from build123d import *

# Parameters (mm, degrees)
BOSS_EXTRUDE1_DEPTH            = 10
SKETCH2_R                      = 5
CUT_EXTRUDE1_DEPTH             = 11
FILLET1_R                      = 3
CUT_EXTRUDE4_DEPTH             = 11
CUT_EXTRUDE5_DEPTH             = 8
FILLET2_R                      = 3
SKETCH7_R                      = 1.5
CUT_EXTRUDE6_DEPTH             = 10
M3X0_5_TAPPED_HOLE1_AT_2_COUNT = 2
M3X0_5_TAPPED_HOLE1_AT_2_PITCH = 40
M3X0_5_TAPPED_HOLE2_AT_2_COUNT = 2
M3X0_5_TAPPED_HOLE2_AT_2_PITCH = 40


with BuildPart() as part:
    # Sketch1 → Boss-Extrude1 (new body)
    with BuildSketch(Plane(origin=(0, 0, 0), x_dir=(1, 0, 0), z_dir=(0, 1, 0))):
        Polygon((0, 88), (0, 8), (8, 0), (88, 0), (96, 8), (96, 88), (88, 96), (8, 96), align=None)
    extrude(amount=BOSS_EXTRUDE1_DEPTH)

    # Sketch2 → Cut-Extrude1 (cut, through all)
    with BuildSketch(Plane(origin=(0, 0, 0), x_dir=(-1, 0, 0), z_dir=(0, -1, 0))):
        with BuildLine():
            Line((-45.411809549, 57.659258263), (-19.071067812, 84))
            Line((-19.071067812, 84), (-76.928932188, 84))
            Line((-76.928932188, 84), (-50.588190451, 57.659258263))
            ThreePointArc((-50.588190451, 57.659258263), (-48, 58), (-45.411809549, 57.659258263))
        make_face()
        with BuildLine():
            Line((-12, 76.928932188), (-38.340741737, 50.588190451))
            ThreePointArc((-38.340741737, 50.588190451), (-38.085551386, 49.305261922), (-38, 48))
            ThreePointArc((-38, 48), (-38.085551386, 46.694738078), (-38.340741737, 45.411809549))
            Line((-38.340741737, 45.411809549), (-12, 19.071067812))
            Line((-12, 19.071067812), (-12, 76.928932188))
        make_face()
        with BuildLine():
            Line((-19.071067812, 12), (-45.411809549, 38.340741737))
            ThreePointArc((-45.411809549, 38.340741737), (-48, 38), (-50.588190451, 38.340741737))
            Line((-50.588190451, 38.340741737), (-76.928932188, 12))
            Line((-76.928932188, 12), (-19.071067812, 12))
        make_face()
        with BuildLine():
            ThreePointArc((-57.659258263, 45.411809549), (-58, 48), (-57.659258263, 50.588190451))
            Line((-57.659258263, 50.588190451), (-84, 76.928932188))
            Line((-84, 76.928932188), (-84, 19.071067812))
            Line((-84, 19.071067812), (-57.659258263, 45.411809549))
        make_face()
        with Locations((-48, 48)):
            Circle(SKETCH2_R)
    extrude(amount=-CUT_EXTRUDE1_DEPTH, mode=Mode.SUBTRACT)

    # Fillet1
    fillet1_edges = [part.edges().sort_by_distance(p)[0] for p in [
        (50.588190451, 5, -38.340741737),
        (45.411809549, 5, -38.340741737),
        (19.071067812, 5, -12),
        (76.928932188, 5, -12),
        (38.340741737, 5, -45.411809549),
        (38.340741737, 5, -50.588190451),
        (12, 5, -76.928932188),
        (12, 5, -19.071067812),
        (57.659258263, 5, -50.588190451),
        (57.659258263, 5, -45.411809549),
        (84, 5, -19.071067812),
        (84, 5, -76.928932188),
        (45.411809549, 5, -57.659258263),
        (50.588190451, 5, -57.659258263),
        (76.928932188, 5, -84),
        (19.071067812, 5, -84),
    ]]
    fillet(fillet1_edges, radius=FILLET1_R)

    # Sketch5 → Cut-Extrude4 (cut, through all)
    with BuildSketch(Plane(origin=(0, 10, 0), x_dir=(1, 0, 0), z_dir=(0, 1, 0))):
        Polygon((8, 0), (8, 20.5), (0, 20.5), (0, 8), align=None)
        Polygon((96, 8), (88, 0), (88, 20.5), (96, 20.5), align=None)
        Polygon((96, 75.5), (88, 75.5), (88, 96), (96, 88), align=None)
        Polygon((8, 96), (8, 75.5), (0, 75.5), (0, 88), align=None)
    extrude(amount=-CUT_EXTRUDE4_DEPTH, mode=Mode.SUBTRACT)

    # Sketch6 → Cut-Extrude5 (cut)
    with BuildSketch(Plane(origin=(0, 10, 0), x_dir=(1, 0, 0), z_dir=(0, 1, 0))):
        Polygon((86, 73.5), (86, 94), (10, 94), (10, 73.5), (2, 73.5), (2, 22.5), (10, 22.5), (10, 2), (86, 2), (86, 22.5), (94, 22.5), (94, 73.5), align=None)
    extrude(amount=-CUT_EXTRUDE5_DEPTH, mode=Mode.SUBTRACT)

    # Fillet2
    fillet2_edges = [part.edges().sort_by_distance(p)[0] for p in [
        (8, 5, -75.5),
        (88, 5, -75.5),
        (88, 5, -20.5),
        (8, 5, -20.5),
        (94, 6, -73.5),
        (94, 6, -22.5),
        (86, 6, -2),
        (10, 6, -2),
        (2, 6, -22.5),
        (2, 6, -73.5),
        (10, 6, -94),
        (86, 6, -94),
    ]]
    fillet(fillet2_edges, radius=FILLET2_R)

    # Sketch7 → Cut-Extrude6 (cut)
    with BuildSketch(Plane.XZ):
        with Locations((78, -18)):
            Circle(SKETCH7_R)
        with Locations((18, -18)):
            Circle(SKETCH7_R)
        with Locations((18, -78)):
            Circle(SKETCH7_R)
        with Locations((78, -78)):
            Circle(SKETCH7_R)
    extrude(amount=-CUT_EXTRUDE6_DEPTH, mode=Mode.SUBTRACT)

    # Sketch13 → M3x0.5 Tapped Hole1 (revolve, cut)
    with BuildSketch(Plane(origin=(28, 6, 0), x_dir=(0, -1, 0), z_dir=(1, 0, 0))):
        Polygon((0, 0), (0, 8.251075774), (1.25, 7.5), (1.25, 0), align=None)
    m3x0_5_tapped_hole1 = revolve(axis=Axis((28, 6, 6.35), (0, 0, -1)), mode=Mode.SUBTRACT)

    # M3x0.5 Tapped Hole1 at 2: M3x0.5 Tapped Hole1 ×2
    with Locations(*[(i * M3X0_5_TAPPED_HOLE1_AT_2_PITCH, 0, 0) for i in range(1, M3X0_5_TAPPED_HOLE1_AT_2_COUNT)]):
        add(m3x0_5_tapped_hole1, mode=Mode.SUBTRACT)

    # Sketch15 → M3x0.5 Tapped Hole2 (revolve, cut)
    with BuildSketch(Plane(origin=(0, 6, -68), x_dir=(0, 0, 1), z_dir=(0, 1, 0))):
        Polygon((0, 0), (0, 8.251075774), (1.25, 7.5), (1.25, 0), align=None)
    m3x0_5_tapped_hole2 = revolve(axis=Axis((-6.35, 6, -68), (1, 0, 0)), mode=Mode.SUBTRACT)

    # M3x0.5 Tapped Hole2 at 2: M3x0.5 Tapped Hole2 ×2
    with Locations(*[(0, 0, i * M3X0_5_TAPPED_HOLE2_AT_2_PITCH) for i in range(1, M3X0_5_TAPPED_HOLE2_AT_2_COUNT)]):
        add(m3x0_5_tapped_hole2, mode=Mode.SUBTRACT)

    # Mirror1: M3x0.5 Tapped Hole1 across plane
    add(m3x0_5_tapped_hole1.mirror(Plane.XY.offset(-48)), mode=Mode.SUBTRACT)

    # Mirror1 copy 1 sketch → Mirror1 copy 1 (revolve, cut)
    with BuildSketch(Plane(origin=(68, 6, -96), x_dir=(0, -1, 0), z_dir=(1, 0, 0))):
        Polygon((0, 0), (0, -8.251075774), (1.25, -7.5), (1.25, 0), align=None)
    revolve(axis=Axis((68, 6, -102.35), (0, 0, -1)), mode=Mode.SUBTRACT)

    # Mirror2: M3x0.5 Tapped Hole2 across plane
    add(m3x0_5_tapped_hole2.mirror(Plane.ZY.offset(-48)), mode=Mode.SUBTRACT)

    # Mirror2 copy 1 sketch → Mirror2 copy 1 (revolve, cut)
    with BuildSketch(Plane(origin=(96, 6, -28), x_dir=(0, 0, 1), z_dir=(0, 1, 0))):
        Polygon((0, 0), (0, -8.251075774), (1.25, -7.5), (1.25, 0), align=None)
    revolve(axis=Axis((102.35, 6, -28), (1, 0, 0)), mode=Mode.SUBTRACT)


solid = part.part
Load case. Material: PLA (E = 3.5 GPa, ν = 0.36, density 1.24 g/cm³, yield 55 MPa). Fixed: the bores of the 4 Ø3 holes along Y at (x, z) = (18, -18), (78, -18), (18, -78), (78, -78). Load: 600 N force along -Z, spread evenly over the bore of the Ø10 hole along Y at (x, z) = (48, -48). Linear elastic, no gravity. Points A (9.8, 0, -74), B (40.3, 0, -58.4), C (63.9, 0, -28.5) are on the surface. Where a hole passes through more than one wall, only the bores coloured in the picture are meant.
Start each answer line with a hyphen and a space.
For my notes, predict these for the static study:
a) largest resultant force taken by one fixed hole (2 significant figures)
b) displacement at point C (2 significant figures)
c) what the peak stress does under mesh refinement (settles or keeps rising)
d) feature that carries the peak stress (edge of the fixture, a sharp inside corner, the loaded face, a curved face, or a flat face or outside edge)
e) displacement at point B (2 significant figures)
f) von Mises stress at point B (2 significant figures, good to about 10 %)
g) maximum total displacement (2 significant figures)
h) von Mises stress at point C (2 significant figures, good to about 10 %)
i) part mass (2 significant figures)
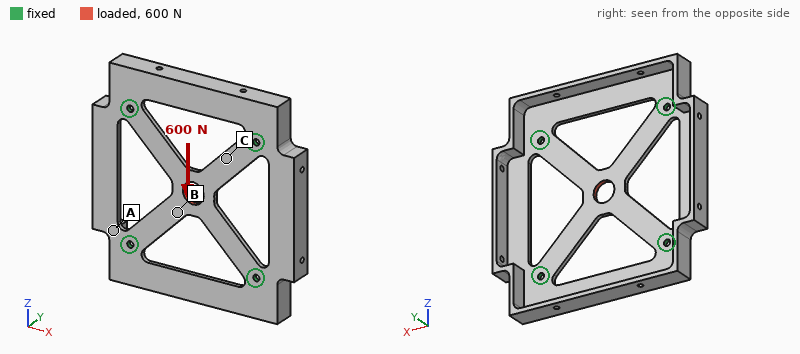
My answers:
- 200 N
- 0.078 mm
- keeps rising
- edge of the fixture
- 0.13 mm
- 9.1 MPa
- 0.18 mm
- 11 MPa
- 21 g
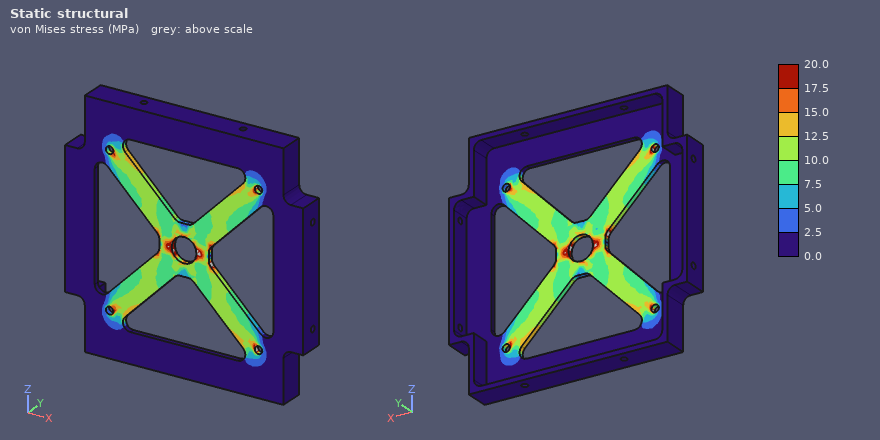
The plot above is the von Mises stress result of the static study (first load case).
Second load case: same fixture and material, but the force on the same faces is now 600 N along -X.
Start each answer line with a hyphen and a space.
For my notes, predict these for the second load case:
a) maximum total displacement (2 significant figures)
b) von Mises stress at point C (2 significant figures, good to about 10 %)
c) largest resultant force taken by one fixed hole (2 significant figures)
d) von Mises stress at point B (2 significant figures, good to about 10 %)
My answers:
- 0.18 mm
- 9.6 MPa
- 200 N
- 10 MPa
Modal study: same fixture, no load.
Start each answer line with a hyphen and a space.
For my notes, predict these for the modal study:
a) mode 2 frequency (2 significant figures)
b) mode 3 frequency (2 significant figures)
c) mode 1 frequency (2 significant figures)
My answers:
- 770 Hz
- 840 Hz
- 580 Hz
